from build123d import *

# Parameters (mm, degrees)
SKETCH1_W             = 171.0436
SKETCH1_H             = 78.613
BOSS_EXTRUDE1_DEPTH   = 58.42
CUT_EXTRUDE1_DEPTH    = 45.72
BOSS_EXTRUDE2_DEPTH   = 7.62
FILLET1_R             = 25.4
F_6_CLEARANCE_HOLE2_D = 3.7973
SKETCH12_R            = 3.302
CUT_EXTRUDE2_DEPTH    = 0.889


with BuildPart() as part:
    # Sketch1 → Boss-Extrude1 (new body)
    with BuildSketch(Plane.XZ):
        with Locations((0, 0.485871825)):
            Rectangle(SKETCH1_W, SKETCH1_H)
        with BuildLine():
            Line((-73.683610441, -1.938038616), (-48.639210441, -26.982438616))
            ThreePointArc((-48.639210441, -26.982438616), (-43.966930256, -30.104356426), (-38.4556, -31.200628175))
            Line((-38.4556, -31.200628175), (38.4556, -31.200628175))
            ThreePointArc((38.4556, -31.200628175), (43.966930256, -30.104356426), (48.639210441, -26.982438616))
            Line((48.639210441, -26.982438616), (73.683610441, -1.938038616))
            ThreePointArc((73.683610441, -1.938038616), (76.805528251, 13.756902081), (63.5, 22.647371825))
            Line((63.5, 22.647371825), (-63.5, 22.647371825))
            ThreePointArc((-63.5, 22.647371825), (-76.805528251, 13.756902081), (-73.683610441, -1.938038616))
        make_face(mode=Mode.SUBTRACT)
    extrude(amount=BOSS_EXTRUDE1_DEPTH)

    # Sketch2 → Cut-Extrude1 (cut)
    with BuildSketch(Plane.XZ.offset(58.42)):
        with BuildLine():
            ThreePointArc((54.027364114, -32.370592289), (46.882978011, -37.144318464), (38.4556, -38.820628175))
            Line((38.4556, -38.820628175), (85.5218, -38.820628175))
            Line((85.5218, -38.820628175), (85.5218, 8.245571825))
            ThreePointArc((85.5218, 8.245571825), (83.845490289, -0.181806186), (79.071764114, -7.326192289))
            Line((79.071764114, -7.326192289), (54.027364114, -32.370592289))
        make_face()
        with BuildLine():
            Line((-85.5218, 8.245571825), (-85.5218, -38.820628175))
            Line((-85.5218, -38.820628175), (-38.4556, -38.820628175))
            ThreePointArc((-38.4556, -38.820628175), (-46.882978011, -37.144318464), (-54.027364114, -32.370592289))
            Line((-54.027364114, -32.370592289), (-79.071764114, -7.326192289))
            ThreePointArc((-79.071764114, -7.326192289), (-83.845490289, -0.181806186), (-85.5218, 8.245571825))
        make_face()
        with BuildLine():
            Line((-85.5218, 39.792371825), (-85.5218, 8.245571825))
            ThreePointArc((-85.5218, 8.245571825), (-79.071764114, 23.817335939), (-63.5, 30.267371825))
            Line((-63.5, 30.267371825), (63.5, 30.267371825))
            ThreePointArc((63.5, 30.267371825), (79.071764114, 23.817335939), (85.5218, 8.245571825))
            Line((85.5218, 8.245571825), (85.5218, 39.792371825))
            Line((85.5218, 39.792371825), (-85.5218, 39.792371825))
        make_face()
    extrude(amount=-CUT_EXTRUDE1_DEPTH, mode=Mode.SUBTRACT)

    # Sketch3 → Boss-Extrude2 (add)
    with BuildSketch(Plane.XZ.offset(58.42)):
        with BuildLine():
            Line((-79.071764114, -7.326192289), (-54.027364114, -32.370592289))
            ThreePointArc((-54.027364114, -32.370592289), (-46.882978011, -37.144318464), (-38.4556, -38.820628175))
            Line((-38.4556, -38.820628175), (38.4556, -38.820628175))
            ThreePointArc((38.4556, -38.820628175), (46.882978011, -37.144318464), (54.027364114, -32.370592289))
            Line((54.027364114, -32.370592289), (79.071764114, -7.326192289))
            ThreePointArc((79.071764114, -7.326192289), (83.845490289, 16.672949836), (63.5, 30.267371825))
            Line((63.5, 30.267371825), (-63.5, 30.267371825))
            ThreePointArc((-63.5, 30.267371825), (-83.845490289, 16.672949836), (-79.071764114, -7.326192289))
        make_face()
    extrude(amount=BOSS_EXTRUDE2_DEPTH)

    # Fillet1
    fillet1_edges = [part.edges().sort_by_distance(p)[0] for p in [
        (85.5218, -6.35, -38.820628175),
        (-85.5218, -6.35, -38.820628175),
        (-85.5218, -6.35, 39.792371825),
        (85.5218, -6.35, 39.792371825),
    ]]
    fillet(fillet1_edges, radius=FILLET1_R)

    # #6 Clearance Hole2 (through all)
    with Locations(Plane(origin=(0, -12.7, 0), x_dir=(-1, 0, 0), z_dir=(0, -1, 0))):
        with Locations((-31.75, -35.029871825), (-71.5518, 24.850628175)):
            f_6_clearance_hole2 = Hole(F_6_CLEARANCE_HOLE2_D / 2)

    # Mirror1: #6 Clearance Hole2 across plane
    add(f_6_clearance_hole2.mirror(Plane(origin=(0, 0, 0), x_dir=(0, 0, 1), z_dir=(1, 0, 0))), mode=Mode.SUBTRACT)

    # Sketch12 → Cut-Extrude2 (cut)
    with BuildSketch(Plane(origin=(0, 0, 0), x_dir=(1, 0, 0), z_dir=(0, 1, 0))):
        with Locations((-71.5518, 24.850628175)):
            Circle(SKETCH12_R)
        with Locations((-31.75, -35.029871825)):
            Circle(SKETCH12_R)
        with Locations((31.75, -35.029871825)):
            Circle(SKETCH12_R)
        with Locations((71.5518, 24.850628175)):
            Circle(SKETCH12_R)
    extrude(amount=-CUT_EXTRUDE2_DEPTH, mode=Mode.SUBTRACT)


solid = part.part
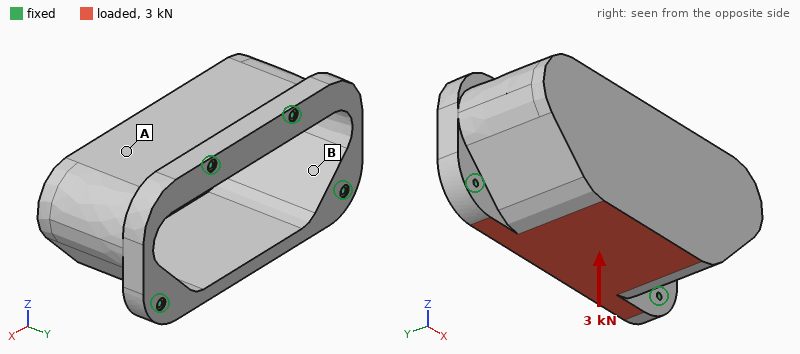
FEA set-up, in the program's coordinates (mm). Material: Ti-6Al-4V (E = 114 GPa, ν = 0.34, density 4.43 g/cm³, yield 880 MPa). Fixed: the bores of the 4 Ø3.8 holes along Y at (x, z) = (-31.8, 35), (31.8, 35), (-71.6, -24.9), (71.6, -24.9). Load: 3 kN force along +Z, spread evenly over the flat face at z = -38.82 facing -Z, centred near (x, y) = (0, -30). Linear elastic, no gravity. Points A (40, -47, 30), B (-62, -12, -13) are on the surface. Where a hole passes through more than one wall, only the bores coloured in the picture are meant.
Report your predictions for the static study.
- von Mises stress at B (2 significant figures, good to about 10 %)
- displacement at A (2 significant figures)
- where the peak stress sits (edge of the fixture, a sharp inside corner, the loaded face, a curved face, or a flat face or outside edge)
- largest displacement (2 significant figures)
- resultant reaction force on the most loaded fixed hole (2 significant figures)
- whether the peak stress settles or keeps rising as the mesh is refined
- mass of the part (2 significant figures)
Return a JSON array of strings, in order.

["7.9 MPa", "7.4 µm", "edge of the fixture", "44 µm", "1.9 kN", "keeps rising", "1.3 kg"]
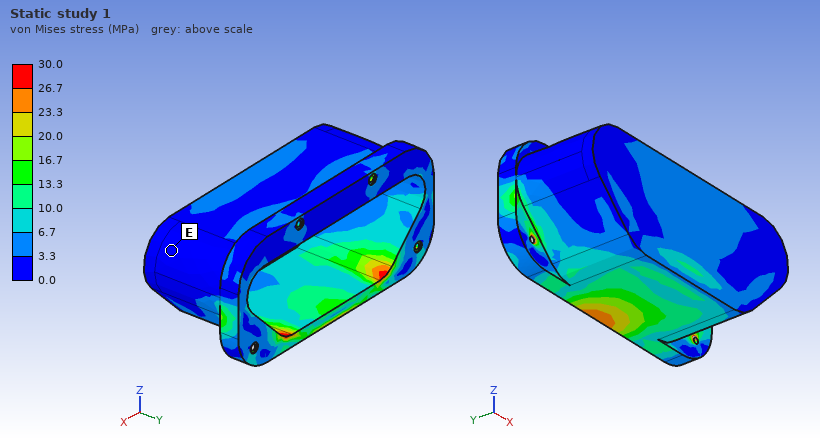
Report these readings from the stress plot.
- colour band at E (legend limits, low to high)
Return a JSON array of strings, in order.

["0.0 to 3.3 MPa"]
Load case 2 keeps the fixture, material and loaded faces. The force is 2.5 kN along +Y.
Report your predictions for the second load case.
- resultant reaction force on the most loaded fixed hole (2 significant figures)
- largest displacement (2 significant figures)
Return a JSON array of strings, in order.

["1.7 kN", "12 µm"]
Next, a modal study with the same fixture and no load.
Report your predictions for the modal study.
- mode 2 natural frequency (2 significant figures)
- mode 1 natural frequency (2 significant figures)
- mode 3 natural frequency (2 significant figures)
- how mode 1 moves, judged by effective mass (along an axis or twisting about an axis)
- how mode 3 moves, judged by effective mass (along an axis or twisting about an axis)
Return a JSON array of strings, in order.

["4100 Hz", "2500 Hz", "4300 Hz", "along Z", "along X"]
